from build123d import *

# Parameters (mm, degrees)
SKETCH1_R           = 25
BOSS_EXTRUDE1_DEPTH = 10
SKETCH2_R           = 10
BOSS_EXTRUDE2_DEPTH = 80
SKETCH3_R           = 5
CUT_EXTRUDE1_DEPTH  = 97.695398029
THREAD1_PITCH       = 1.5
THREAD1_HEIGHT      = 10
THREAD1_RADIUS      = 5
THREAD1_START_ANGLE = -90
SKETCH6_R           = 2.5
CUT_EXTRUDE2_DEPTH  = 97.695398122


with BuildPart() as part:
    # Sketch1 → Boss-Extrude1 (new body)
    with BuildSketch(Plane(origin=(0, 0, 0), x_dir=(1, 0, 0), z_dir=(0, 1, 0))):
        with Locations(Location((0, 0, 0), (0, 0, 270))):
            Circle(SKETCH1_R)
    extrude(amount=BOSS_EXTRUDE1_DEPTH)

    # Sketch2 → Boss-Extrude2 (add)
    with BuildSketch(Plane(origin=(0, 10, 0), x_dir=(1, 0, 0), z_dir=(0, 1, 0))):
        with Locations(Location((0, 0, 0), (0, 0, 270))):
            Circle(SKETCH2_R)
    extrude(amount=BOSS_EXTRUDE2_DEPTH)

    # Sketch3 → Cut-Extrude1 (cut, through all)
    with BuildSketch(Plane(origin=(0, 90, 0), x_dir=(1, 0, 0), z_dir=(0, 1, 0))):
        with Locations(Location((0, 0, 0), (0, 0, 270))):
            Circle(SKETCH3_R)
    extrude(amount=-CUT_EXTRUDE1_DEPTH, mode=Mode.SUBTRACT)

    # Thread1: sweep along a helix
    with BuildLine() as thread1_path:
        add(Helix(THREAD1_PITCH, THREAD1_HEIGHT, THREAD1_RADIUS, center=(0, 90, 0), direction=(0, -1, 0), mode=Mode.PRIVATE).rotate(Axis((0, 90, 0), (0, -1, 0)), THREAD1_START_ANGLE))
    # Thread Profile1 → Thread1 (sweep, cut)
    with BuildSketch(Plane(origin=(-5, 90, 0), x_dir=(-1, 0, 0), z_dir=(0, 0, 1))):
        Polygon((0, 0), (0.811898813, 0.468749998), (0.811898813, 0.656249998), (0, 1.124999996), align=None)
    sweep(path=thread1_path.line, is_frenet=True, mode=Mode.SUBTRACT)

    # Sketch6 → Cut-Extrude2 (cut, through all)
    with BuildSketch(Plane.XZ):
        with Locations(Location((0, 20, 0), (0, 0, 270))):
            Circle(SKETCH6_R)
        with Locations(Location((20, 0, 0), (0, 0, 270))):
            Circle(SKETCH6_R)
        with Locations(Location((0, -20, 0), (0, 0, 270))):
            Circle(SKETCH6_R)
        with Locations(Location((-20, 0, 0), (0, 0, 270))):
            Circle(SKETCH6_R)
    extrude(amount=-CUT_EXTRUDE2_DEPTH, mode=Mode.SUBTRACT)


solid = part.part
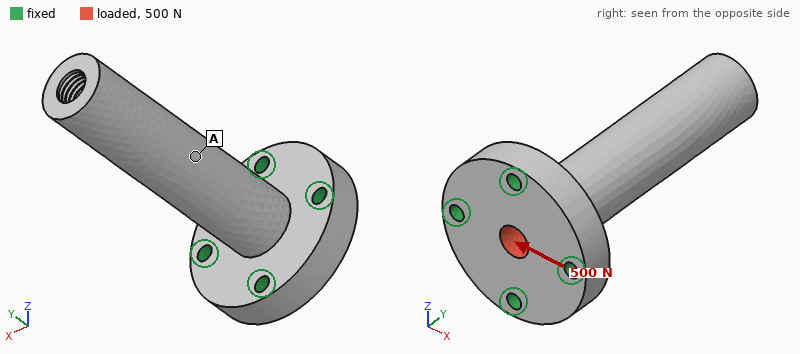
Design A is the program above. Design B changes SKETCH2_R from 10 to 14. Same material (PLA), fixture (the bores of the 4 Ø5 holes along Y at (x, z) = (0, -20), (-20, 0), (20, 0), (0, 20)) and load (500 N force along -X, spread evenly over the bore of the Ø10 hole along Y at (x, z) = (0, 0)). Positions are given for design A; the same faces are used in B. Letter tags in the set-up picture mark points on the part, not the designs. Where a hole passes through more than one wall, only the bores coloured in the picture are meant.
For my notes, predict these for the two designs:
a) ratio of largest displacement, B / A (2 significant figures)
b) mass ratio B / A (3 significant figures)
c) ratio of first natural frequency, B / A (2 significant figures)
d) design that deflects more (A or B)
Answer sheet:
0.29
1.66
1.2
A
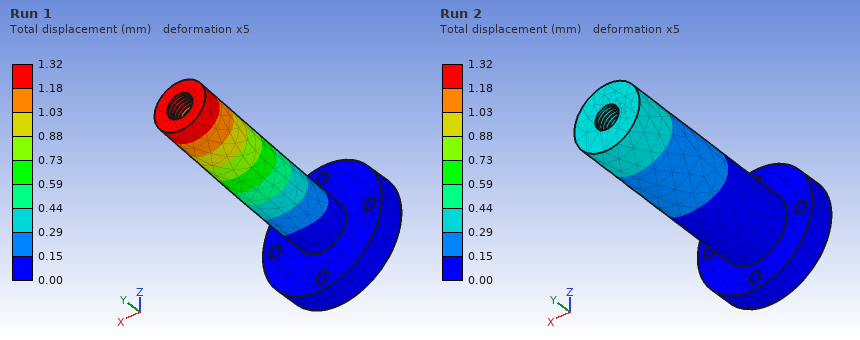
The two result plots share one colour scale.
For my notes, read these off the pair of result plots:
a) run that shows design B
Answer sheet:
Run 2
